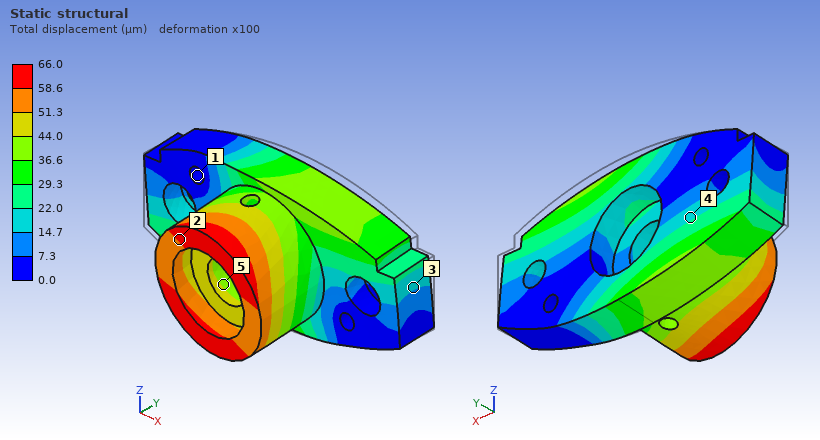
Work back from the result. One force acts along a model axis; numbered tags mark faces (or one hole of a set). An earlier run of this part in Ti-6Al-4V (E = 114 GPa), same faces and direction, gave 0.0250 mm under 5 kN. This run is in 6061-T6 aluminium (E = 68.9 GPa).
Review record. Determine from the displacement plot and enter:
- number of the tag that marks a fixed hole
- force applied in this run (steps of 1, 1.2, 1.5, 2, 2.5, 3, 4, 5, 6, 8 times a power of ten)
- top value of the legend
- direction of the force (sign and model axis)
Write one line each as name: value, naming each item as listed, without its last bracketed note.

number of the tag that marks a fixed hole: 1
force applied in this run: 8 kN
top value of the legend: 66.0 µm
direction of the force: -Z
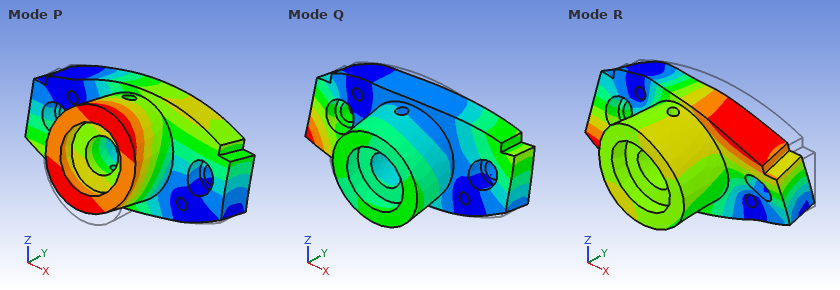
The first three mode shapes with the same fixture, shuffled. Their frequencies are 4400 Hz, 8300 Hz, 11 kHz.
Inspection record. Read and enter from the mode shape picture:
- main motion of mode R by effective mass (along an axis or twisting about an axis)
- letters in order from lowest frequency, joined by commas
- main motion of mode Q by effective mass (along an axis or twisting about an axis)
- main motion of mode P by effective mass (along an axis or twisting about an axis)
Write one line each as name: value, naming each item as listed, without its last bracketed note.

main motion of mode R by effective mass: along Y
letters in order from lowest frequency, joined by commas: P, R, Q
main motion of mode Q by effective mass: along Z
main motion of mode P by effective mass: along Z
